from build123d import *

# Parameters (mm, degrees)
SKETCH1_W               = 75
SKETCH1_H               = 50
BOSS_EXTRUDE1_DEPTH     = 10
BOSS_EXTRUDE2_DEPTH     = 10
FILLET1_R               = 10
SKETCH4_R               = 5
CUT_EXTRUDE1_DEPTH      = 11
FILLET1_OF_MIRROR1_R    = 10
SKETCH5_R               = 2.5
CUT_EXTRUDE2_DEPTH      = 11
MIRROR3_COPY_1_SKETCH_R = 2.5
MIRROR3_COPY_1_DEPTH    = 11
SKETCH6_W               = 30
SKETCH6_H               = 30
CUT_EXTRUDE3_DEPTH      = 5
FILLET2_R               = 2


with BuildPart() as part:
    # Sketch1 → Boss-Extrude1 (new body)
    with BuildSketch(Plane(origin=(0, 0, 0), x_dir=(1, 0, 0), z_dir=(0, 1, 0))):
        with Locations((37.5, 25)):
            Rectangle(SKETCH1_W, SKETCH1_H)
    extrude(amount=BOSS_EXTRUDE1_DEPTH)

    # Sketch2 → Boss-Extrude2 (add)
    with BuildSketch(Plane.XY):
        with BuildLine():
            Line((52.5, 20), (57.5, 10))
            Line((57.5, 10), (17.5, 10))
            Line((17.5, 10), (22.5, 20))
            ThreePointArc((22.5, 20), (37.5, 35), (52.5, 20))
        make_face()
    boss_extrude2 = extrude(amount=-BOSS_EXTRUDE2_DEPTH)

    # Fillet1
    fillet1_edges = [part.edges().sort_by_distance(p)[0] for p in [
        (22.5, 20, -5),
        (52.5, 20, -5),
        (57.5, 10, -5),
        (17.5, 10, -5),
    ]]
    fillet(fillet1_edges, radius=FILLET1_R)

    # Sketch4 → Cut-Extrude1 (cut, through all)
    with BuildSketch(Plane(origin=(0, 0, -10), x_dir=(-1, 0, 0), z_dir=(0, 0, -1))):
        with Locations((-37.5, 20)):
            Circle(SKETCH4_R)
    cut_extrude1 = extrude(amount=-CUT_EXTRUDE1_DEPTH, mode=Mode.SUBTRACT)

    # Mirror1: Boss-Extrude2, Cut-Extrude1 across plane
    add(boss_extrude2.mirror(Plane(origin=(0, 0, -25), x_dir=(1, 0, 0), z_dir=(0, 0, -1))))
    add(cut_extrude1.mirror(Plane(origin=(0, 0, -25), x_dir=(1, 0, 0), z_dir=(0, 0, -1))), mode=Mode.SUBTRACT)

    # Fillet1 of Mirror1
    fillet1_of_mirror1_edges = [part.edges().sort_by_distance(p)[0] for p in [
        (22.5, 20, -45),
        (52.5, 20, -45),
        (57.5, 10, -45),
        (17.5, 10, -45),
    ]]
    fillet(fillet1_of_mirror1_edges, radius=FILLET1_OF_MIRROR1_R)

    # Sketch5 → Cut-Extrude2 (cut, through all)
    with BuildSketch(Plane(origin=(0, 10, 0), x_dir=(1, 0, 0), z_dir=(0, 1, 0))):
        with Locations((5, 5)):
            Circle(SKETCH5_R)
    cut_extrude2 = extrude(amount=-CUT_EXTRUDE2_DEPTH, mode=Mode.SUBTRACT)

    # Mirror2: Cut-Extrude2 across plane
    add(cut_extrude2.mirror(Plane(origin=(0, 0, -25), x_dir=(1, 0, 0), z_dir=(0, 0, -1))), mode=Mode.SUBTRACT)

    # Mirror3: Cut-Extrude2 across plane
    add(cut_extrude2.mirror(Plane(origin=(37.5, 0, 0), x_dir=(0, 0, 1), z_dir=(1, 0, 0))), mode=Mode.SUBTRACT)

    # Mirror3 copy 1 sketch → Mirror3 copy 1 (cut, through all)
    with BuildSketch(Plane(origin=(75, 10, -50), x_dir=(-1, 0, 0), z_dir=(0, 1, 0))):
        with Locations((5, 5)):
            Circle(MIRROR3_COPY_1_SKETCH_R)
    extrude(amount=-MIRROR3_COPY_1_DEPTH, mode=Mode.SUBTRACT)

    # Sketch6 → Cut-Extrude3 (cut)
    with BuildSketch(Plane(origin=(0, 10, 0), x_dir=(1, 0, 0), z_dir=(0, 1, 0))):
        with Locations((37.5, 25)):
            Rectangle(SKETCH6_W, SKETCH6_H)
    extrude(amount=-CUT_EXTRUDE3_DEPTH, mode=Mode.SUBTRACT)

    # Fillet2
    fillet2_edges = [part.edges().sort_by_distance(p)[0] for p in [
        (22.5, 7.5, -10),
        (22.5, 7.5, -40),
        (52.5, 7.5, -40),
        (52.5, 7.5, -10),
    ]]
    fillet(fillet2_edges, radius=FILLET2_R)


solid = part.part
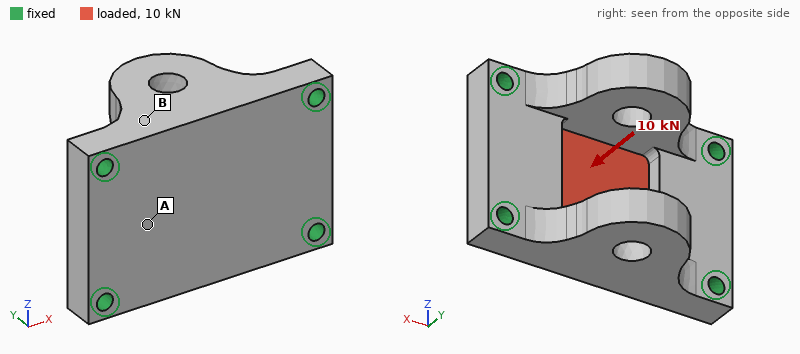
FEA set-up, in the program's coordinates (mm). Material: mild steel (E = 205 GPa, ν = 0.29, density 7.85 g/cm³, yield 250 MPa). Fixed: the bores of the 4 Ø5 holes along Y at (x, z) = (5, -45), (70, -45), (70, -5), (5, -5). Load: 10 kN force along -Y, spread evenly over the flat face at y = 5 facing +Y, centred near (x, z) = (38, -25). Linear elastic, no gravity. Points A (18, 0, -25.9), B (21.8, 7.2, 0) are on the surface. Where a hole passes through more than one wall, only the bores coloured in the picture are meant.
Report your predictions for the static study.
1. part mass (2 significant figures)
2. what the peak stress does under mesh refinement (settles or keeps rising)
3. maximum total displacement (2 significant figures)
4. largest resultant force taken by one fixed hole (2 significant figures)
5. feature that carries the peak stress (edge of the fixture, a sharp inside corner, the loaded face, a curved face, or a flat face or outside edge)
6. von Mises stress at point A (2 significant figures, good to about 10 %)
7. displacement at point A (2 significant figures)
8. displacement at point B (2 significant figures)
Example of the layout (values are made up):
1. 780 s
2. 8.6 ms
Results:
1. 350 g
2. keeps rising
3. 31 µm
4. 2.5 kN
5. edge of the fixture
6. 39 MPa
7. 13 µm
8. 5.3 µm
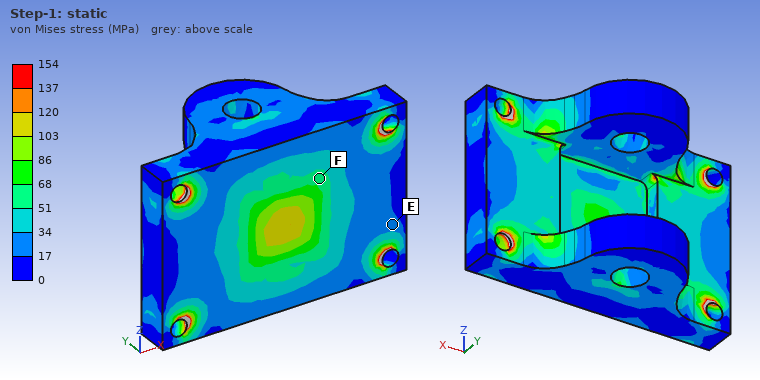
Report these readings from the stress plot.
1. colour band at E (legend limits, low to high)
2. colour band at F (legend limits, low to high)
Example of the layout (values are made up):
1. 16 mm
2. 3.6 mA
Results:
1. 17 to 34 MPa
2. 51 to 68 MPa
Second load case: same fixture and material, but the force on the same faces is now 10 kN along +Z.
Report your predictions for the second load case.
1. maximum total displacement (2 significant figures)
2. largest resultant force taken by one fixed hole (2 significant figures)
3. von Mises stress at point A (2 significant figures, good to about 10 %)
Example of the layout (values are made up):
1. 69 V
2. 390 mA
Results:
1. 6.5 µm
2. 3.1 kN
3. 20 MPa
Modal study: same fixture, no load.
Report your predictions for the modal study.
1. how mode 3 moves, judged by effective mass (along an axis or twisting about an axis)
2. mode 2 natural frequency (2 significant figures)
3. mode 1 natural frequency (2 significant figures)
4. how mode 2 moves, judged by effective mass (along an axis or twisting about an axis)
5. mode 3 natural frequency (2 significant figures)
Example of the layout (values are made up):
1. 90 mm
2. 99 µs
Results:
1. along Y
2. 7100 Hz
3. 6700 Hz
4. along Z
5. 10 kHz
